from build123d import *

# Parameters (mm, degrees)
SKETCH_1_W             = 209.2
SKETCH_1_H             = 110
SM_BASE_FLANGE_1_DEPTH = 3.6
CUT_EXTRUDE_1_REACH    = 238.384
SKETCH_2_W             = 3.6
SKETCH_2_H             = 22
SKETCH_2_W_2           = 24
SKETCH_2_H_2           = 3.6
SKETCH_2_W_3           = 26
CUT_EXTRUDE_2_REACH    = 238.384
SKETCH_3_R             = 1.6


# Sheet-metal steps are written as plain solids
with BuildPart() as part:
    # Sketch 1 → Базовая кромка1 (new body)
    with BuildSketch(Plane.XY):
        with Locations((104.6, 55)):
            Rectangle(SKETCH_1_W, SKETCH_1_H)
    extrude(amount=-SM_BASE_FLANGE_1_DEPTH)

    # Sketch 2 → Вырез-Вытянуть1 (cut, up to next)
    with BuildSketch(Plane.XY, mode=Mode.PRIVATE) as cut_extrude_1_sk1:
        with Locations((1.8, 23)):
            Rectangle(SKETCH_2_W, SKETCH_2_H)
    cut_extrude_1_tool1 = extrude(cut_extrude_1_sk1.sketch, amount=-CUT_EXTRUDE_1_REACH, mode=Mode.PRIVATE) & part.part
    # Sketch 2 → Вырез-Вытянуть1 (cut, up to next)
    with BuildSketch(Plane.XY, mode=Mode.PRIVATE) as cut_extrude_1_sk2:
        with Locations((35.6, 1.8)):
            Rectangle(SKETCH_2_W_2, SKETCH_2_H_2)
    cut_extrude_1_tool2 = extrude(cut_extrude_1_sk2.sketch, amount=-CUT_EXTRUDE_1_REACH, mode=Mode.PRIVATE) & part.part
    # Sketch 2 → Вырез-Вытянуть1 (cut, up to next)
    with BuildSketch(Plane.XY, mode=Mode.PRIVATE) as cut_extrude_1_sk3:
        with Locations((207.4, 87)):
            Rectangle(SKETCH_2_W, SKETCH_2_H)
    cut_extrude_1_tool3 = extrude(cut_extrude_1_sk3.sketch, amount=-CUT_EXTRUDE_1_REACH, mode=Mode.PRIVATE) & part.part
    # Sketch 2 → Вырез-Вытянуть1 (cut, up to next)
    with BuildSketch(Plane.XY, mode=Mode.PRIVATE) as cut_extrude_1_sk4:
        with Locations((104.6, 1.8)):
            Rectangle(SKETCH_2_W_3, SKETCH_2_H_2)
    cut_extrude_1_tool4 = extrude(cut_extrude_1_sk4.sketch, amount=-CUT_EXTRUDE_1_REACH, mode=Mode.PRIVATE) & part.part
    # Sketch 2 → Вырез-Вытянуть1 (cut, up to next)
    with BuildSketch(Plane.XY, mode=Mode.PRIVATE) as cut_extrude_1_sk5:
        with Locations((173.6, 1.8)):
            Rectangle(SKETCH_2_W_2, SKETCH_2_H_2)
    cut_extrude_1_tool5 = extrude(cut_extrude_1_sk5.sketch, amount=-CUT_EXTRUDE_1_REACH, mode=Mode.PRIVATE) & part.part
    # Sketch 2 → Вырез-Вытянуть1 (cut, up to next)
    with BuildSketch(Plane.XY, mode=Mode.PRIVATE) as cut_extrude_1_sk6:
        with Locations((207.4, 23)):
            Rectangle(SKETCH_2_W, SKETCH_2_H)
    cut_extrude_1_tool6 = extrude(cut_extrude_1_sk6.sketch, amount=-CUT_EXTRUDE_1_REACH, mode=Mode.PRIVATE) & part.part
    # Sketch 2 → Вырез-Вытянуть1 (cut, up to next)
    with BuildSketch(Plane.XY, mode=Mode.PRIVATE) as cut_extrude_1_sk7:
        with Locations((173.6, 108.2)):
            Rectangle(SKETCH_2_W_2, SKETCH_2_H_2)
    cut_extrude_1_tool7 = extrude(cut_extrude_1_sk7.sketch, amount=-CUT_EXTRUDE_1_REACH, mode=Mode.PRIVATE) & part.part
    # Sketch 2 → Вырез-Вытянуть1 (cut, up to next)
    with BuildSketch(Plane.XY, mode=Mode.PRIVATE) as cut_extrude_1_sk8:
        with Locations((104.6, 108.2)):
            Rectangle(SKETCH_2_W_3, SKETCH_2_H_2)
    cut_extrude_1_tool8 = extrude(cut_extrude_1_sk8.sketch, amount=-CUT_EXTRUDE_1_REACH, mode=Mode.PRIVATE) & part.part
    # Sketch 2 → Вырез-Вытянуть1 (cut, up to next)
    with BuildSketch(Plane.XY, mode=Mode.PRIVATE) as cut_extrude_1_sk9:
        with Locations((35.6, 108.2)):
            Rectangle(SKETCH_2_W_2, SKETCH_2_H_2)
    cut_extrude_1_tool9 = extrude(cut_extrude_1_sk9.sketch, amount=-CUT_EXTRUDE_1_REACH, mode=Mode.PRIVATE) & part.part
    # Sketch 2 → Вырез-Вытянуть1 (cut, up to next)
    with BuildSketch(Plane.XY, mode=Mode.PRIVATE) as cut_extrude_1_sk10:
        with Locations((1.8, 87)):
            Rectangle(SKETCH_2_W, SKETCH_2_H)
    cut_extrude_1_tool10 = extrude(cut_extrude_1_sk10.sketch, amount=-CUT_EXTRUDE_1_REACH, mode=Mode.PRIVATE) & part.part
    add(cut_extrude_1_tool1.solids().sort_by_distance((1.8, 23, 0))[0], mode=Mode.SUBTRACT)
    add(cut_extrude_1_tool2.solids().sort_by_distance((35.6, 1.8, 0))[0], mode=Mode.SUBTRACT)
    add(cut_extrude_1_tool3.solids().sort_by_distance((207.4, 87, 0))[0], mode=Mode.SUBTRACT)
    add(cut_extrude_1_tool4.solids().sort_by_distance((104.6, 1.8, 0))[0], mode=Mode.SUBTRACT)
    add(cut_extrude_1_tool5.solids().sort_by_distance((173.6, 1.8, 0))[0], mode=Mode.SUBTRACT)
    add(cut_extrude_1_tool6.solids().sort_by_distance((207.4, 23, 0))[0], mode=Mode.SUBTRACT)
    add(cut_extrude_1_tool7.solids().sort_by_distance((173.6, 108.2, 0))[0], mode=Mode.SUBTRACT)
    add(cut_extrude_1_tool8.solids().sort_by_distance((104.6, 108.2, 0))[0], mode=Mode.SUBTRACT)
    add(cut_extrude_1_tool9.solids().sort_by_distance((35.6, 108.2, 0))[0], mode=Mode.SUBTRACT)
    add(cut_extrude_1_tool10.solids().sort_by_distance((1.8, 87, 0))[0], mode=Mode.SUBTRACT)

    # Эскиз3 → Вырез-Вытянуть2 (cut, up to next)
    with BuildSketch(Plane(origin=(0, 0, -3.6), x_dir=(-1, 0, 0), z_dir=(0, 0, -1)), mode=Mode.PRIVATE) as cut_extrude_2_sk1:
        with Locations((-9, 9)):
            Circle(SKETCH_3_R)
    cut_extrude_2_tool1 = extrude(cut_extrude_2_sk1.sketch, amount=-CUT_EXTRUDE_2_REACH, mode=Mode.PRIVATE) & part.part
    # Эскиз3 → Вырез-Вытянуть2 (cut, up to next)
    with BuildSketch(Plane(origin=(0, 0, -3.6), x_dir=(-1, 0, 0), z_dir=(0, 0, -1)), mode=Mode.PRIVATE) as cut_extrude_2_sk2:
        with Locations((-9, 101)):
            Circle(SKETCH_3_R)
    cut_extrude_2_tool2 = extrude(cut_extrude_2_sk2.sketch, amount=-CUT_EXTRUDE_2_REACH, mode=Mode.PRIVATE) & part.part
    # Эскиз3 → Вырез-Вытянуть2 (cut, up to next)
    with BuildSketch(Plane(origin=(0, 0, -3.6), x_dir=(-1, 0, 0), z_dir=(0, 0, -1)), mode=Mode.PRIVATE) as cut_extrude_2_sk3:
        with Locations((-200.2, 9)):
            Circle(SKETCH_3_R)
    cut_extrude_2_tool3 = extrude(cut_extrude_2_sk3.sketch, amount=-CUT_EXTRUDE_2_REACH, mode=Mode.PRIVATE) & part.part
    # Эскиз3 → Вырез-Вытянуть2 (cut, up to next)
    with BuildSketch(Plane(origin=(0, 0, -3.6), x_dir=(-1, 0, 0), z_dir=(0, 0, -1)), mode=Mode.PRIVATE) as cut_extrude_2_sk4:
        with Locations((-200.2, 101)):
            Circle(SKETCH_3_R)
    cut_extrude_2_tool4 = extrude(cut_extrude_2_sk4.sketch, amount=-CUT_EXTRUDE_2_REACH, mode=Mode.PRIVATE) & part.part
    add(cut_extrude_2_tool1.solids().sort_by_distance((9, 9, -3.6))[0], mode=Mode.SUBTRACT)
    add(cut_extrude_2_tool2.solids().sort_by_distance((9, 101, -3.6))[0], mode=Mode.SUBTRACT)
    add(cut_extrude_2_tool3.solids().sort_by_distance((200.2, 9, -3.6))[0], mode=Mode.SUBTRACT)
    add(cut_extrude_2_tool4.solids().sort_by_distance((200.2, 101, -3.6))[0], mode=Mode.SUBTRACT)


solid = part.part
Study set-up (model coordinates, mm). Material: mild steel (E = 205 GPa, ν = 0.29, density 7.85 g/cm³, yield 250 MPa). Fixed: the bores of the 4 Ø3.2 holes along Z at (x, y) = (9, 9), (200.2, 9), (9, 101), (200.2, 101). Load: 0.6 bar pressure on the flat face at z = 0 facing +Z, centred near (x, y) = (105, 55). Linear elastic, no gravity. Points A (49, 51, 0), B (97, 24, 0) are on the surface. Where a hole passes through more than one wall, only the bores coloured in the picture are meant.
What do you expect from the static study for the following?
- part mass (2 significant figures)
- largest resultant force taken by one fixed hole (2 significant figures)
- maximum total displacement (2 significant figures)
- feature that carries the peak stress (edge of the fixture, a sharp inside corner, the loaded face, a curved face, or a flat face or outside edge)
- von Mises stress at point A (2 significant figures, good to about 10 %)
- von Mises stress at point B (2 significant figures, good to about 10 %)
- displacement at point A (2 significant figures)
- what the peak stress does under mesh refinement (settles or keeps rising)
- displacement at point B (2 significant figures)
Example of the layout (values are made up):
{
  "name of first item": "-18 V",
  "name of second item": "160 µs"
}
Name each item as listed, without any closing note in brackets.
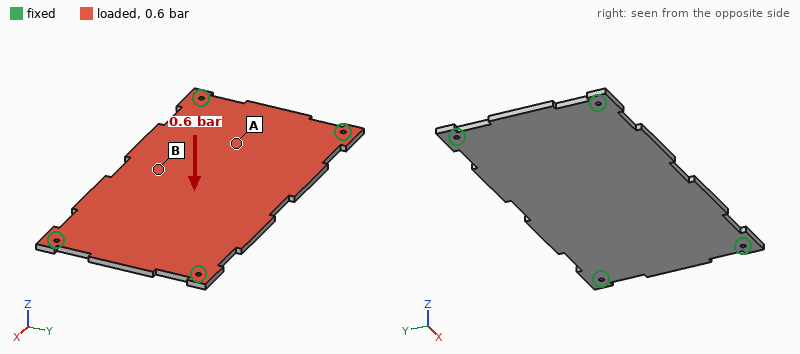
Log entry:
{
  "part mass": "630 g",
  "largest resultant force taken by one fixed hole": "330 N",
  "maximum total displacement": "0.41 mm",
  "feature that carries the peak stress": "edge of the fixture",
  "von Mises stress at point A": "17 MPa",
  "von Mises stress at point B": "52 MPa",
  "displacement at point A": "0.23 mm",
  "what the peak stress does under mesh refinement": "keeps rising",
  "displacement at point B": "0.40 mm"
}
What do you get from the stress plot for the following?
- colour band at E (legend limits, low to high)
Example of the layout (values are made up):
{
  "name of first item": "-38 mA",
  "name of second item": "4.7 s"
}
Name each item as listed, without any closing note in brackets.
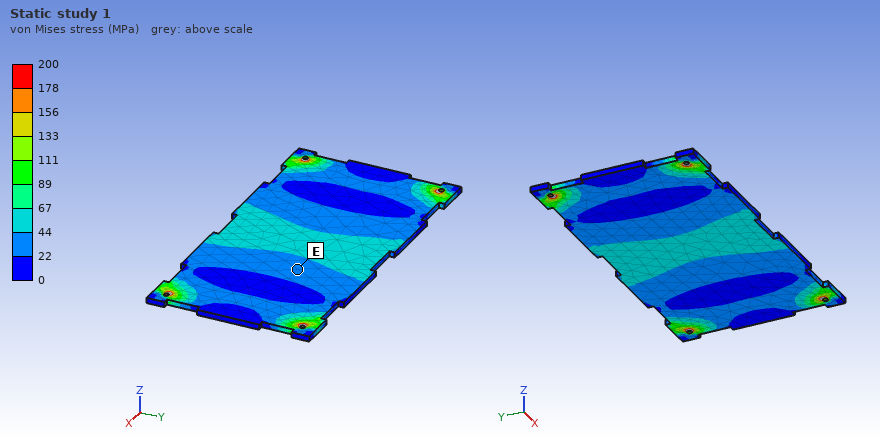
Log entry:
{
  "colour band at E": "22 to 44 MPa"
}
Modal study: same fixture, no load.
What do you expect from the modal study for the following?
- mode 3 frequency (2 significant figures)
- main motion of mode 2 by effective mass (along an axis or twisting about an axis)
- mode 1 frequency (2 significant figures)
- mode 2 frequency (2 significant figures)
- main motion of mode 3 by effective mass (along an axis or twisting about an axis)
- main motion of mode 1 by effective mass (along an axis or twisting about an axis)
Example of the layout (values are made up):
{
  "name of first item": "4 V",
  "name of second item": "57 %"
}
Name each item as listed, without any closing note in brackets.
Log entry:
{
  "mode 3 frequency": "1200 Hz",
  "main motion of mode 2 by effective mass": "twisting about X",
  "mode 1 frequency": "410 Hz",
  "mode 2 frequency": "770 Hz",
  "main motion of mode 3 by effective mass": "twisting about Y",
  "main motion of mode 1 by effective mass": "along Z"
}
